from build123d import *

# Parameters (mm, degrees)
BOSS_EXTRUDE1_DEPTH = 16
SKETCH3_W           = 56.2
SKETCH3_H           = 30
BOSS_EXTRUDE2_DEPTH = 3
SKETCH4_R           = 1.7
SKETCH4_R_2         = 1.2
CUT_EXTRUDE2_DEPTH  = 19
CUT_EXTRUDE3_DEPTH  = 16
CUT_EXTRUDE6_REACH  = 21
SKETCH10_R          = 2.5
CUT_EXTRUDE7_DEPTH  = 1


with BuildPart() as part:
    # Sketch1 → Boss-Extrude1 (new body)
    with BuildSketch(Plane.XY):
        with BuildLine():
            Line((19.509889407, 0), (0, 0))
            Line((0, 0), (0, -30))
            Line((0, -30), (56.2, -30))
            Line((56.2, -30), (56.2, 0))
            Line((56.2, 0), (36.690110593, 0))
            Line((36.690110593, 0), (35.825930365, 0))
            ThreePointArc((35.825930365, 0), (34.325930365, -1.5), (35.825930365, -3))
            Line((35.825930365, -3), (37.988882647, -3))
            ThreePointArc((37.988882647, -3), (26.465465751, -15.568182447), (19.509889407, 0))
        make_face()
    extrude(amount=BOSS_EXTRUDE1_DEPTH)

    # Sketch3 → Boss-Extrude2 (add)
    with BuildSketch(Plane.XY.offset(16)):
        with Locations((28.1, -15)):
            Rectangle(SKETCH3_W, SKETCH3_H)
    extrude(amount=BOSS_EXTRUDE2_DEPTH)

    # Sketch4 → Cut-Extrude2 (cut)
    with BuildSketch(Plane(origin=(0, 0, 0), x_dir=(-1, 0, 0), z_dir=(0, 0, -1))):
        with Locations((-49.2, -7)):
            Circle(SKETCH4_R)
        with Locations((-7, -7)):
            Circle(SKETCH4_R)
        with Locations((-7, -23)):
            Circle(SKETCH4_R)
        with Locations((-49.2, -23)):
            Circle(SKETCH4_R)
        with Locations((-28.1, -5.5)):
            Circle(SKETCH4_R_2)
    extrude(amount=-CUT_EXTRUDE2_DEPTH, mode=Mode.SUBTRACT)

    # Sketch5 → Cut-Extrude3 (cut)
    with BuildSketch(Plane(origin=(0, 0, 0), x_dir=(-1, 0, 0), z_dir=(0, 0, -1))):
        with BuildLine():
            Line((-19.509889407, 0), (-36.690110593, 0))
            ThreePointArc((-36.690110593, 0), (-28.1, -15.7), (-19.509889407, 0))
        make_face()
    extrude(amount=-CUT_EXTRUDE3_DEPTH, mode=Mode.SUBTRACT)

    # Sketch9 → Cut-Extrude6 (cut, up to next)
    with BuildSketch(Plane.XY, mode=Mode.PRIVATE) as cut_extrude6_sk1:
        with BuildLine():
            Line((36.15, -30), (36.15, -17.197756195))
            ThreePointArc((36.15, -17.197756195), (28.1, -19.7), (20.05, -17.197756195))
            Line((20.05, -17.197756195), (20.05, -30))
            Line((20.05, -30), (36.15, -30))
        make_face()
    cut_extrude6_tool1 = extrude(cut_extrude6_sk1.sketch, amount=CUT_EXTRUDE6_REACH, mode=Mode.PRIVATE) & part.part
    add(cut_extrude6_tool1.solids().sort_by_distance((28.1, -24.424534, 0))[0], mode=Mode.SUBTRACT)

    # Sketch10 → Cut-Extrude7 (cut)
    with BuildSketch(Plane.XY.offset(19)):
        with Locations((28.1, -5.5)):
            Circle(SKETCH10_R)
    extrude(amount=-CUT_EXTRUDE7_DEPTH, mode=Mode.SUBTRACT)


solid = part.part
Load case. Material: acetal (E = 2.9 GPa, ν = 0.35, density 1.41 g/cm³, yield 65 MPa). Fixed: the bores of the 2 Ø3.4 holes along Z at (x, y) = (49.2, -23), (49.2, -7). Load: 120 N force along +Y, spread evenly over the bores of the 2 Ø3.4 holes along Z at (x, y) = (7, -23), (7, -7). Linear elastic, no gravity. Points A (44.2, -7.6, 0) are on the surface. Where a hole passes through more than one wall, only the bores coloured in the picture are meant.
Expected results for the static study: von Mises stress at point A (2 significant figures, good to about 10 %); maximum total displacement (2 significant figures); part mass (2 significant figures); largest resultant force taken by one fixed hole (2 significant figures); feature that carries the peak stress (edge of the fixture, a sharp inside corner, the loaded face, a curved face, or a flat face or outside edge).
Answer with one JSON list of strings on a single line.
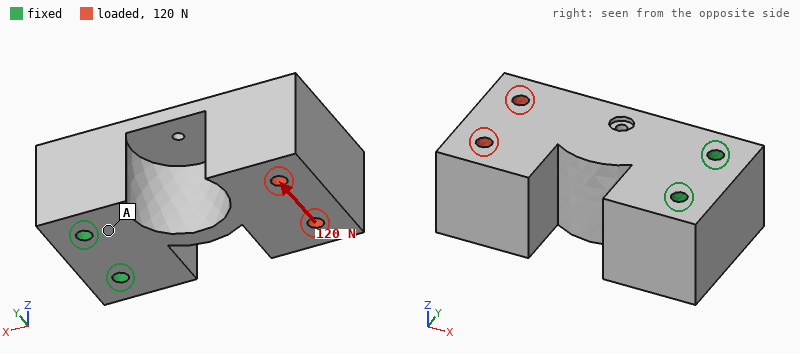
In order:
["1.9 MPa", "0.63 mm", "33 g", "300 N", "a curved face"]
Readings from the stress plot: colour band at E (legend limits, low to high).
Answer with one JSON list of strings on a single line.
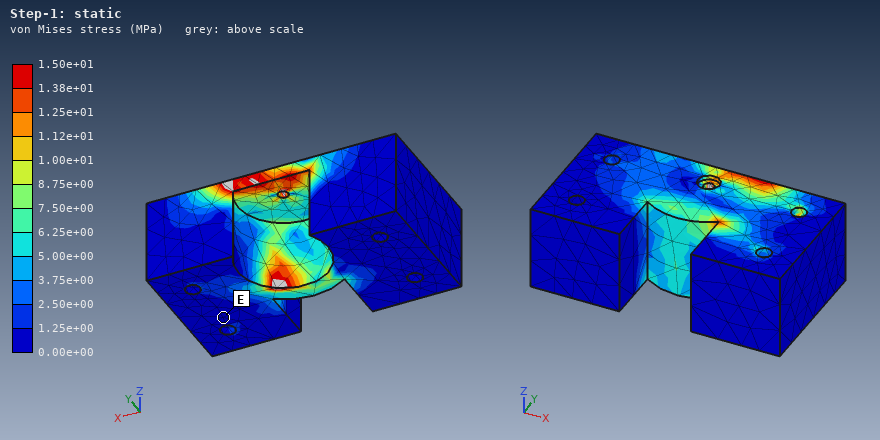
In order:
["0.00e+00 to 1.25e+00 MPa"]
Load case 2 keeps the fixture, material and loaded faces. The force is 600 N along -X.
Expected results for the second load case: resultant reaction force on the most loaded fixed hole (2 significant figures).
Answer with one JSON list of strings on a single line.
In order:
["320 N"]
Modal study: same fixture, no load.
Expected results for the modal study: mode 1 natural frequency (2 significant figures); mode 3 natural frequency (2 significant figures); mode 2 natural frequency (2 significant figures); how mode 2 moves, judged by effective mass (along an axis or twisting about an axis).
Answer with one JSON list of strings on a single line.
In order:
["670 Hz", "1400 Hz", "870 Hz", "along Z"]
